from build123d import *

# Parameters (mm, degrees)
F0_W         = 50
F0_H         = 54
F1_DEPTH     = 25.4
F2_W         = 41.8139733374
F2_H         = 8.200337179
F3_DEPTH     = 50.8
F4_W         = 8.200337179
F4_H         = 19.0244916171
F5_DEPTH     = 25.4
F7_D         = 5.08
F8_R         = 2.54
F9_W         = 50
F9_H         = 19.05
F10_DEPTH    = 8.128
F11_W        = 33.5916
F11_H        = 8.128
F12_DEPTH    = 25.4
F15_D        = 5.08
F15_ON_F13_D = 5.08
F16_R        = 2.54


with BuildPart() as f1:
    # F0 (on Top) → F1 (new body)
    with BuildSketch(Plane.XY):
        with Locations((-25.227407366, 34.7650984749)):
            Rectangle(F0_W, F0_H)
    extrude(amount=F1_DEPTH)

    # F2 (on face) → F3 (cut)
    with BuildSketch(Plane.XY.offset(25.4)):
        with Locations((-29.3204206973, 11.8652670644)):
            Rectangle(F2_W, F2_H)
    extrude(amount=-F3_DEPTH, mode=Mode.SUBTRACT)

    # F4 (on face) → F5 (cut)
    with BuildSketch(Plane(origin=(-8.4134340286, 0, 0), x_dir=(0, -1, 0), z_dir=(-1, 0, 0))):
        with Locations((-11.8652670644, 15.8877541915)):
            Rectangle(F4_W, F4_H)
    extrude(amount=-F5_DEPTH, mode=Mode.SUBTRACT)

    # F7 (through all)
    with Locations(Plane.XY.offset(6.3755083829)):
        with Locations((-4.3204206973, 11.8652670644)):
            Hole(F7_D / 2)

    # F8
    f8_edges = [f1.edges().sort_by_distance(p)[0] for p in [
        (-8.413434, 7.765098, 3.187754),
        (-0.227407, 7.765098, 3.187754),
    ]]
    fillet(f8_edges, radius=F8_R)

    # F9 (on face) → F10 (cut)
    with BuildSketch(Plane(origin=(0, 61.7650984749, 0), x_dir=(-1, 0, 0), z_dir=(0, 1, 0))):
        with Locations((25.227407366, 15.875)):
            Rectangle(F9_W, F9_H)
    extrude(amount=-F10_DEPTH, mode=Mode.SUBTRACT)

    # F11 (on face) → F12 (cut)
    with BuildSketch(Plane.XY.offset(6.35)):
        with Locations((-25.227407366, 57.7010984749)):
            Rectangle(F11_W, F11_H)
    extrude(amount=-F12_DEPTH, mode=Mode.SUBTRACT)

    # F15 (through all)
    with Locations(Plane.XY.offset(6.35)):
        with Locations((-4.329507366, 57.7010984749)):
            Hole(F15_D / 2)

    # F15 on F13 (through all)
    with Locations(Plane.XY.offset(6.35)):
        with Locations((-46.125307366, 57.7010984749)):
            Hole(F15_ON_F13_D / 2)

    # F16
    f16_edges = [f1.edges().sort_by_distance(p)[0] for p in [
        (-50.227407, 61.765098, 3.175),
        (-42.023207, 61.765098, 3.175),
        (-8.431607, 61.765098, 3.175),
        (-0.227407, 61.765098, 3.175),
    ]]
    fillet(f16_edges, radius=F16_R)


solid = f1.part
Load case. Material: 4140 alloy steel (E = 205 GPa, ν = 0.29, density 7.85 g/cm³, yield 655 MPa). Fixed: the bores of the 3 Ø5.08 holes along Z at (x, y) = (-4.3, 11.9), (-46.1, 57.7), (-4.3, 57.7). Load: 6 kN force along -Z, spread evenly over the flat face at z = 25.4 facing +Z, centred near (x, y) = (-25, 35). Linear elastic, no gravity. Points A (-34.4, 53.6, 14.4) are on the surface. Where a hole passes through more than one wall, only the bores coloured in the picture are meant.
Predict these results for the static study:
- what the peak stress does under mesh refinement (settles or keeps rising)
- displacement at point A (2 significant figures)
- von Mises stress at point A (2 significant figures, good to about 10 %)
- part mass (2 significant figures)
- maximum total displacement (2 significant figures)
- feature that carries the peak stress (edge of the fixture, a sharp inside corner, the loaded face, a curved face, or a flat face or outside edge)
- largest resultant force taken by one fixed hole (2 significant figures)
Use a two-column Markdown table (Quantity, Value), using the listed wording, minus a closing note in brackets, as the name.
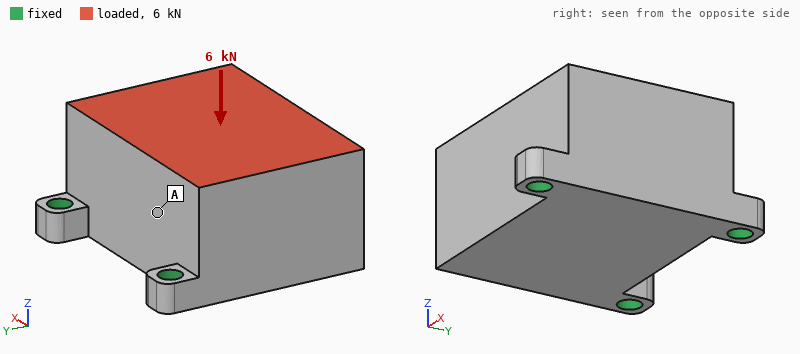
| Quantity | Value |
|---|---|
| what the peak stress does under mesh refinement | keeps rising |
| displacement at point A | 5.7 µm |
| von Mises stress at point A | 17 MPa |
| part mass | 380 g |
| maximum total displacement | 20 µm |
| feature that carries the peak stress | edge of the fixture |
| largest resultant force taken by one fixed hole | 3.2 kN |
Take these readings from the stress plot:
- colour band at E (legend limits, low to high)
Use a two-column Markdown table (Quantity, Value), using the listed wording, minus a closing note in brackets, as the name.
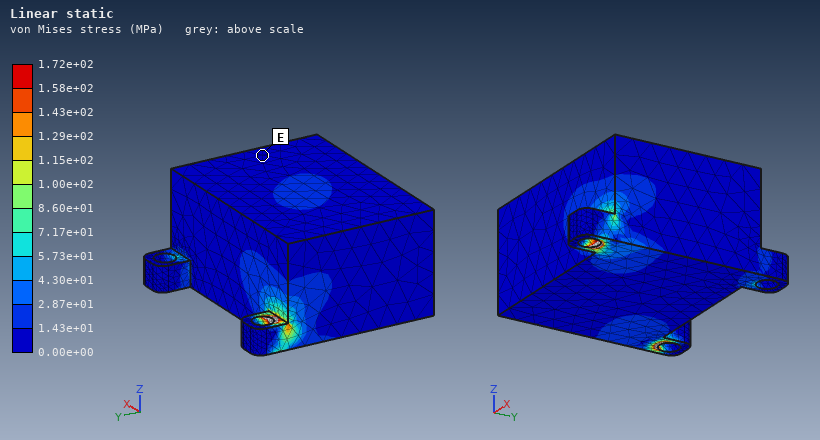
| Quantity | Value |
|---|---|
| colour band at E | 0.00e+00 to 1.43e+01 MPa |
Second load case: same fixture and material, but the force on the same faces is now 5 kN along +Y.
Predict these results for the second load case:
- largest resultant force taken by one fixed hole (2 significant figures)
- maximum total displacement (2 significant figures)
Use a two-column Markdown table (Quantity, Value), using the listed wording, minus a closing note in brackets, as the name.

| Quantity | Value |
|---|---|
| largest resultant force taken by one fixed hole | 3.4 kN |
| maximum total displacement | 21 µm |
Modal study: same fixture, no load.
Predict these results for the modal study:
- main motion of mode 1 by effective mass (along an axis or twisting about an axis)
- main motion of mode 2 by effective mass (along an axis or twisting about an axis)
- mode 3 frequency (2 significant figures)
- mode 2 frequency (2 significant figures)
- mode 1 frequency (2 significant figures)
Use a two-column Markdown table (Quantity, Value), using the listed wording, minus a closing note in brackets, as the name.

| Quantity | Value |
|---|---|
| main motion of mode 1 by effective mass | along Z |
| main motion of mode 2 by effective mass | along X |
| mode 3 frequency | 12 kHz |
| mode 2 frequency | 9500 Hz |
| mode 1 frequency | 5500 Hz |
